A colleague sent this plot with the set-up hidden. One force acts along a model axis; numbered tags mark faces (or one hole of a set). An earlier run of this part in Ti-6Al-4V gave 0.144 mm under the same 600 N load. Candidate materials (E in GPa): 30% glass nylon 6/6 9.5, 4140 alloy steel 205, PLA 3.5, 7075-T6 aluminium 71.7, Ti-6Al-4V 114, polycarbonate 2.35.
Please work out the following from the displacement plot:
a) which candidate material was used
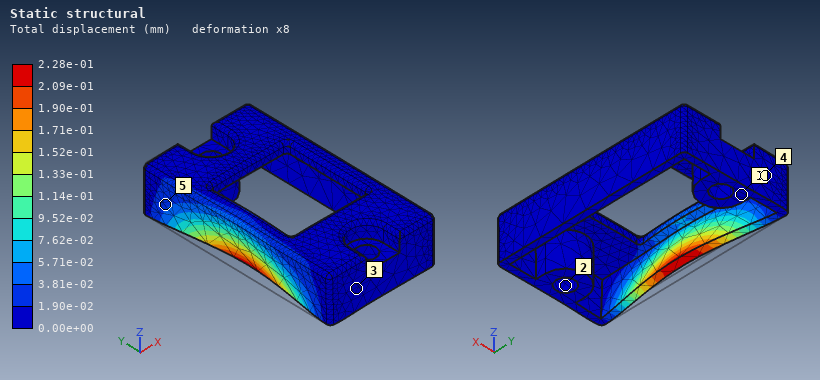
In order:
7075-T6 aluminium
